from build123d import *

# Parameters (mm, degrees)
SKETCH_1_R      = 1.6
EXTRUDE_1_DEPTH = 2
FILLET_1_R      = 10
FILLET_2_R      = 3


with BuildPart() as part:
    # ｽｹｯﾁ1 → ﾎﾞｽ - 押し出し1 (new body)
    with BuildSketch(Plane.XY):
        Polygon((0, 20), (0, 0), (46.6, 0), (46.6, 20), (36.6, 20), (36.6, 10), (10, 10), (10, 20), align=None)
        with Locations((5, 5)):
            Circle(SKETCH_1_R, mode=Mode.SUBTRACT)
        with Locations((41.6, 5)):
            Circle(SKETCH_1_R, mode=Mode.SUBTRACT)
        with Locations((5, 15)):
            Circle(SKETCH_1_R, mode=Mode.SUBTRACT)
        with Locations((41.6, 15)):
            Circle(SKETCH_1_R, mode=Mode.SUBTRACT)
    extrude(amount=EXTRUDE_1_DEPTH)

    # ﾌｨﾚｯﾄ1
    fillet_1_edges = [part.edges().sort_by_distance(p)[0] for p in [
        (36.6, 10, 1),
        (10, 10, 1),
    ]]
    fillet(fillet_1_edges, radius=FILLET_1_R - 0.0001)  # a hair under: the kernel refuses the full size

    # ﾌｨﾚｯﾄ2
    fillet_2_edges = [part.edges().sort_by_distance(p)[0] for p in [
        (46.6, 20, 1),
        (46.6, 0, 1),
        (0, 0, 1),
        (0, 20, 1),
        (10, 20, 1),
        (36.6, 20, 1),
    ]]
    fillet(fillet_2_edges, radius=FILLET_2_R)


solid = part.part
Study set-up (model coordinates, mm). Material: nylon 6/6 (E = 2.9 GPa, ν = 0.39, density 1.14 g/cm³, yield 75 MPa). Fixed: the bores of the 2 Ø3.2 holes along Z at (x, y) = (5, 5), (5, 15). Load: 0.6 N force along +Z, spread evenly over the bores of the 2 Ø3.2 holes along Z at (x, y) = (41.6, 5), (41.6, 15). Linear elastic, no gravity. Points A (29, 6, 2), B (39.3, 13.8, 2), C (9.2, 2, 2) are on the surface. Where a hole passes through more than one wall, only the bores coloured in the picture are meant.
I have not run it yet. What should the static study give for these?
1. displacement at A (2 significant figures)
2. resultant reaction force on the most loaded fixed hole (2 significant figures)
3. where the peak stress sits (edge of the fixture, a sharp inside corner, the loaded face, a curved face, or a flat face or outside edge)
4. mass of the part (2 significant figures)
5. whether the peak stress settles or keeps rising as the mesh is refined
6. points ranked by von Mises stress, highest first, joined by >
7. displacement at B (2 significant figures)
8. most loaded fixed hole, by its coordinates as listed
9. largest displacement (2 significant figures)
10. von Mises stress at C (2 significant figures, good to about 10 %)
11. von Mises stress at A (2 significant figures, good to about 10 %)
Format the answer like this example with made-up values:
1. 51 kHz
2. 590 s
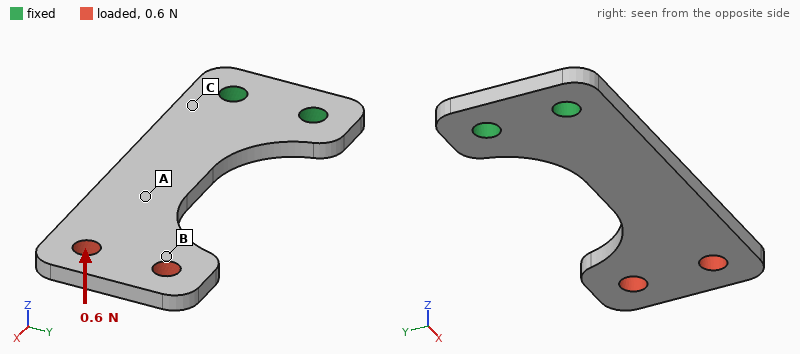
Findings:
1. 0.18 mm
2. 0.48 N
3. edge of the fixture
4. 1.5 g
5. keeps rising
6. C > A > B
7. 0.36 mm
8. (5, 5)
9. 0.49 mm
10. 1.9 MPa
11. 1.2 MPa
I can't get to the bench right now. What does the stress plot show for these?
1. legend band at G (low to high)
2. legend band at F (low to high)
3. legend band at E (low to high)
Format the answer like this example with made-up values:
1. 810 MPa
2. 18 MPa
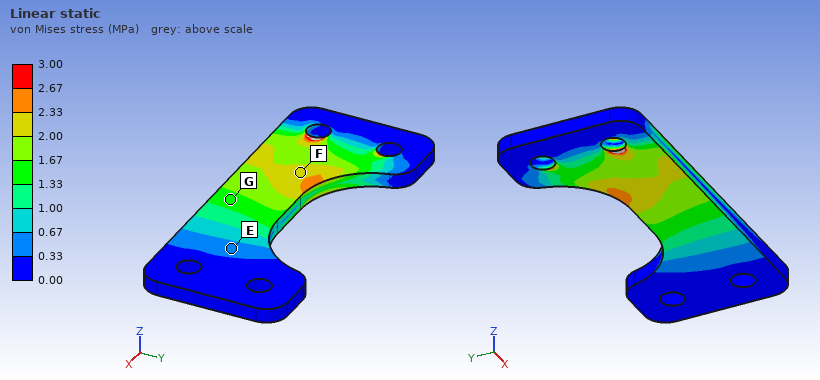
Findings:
1. 1.33 to 1.67 MPa
2. 2.00 to 2.33 MPa
3. 0.33 to 0.67 MPa
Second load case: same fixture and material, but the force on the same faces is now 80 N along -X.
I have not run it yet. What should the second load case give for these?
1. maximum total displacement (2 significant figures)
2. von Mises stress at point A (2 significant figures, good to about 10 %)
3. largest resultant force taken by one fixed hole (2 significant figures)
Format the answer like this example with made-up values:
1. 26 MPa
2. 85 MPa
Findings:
1. 0.51 mm
2. 4.8 MPa
3. 44 N
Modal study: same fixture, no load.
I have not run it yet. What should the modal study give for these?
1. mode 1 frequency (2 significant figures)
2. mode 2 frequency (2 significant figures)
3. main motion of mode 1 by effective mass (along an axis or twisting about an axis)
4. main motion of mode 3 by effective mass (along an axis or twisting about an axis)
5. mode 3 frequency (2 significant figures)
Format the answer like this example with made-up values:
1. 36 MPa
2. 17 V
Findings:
1. 270 Hz
2. 1100 Hz
3. along Z
4. along Y
5. 1400 Hz
